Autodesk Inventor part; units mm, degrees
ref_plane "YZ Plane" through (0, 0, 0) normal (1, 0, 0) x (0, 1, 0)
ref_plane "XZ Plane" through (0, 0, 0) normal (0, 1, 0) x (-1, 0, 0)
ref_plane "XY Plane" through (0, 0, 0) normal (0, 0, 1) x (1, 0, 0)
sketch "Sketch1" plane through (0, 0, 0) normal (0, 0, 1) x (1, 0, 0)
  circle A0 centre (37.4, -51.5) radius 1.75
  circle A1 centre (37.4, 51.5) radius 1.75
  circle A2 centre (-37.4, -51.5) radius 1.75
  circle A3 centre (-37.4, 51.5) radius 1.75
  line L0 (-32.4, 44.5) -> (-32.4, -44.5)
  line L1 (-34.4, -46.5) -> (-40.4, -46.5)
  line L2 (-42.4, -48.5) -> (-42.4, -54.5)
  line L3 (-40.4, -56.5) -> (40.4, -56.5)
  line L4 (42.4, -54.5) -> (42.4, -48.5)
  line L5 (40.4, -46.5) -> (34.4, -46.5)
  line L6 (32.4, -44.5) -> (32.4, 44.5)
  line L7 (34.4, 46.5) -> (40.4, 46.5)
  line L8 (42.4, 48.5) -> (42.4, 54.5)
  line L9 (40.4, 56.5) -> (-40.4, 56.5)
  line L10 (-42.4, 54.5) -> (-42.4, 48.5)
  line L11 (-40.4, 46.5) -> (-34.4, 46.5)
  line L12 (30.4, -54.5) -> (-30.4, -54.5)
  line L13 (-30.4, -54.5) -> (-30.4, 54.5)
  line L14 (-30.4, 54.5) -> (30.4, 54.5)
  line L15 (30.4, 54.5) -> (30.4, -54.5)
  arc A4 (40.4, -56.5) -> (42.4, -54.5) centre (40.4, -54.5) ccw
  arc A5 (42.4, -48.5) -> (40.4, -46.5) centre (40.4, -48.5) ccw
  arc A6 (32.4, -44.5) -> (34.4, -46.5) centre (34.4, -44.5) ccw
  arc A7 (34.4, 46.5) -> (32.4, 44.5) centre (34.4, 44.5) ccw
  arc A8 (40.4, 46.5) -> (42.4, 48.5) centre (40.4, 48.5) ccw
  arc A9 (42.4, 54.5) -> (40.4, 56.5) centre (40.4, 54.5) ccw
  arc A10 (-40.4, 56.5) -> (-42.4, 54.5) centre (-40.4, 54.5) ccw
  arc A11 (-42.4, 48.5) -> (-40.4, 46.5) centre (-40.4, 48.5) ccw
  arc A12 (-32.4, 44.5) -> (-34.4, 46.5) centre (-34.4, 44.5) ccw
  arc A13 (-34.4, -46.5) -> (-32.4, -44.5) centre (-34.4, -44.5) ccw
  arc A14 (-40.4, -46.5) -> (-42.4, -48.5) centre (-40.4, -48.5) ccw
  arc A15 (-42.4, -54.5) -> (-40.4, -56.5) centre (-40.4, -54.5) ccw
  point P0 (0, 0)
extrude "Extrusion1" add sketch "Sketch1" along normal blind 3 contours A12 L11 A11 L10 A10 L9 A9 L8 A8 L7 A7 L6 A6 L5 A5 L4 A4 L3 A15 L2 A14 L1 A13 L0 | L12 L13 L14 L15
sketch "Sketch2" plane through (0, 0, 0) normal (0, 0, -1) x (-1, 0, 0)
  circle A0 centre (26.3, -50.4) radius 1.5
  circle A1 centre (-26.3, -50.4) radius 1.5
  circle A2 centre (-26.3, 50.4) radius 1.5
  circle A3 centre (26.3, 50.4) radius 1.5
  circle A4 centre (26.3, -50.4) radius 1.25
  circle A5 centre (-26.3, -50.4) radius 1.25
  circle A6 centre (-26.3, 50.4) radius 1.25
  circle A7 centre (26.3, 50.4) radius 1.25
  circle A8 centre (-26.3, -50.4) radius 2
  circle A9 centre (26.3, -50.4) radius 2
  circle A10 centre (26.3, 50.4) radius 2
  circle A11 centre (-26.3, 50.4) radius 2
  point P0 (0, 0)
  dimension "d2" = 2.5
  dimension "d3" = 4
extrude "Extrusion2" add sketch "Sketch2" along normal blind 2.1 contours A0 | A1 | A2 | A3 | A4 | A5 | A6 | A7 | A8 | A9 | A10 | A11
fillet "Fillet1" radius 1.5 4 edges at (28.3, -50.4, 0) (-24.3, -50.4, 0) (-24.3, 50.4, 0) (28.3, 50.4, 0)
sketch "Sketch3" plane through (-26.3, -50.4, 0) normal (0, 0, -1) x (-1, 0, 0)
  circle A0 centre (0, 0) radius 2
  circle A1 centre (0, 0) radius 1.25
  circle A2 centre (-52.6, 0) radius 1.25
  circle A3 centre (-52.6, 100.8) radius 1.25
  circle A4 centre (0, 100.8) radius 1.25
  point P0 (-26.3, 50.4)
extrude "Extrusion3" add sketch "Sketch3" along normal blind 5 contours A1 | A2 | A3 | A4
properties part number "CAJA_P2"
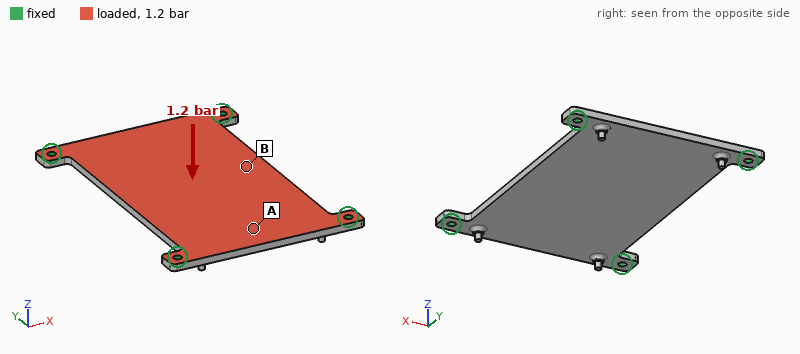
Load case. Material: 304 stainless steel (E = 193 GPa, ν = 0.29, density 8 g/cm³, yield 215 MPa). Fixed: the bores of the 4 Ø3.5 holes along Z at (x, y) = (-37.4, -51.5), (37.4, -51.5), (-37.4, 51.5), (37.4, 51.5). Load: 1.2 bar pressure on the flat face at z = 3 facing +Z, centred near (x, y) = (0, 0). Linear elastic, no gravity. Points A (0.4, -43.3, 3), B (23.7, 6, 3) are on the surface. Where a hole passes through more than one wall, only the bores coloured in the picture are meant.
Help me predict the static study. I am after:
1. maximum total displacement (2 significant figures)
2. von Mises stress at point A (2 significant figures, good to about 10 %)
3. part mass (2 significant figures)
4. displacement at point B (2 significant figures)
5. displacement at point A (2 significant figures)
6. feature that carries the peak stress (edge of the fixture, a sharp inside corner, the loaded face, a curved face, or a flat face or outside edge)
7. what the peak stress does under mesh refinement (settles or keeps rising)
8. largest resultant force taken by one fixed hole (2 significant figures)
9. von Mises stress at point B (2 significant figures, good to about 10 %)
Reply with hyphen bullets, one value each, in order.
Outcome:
- 0.18 mm
- 32 MPa
- 190 g
- 0.17 mm
- 0.076 mm
- edge of the fixture
- keeps rising
- 230 N
- 52 MPa
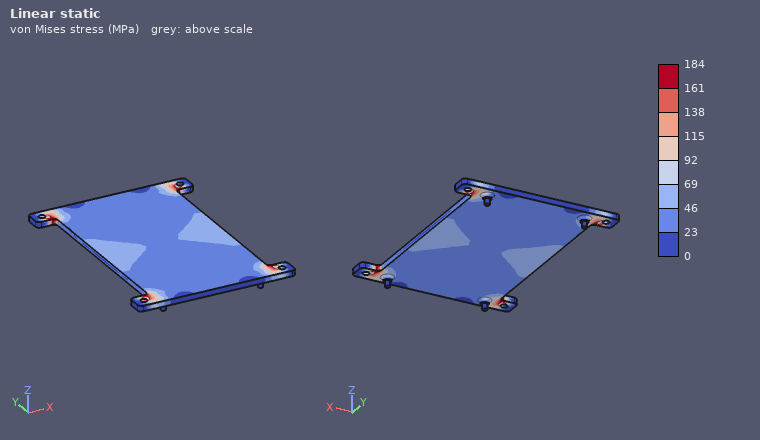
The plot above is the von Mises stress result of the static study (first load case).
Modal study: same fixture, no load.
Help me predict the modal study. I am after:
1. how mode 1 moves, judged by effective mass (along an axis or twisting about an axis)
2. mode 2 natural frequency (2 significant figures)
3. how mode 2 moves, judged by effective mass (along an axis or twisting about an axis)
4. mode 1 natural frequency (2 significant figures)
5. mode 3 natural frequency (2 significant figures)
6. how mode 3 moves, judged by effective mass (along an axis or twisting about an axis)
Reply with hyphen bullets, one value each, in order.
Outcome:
- along Z
- 1900 Hz
- twisting about Y
- 950 Hz
- 2300 Hz
- twisting about X
